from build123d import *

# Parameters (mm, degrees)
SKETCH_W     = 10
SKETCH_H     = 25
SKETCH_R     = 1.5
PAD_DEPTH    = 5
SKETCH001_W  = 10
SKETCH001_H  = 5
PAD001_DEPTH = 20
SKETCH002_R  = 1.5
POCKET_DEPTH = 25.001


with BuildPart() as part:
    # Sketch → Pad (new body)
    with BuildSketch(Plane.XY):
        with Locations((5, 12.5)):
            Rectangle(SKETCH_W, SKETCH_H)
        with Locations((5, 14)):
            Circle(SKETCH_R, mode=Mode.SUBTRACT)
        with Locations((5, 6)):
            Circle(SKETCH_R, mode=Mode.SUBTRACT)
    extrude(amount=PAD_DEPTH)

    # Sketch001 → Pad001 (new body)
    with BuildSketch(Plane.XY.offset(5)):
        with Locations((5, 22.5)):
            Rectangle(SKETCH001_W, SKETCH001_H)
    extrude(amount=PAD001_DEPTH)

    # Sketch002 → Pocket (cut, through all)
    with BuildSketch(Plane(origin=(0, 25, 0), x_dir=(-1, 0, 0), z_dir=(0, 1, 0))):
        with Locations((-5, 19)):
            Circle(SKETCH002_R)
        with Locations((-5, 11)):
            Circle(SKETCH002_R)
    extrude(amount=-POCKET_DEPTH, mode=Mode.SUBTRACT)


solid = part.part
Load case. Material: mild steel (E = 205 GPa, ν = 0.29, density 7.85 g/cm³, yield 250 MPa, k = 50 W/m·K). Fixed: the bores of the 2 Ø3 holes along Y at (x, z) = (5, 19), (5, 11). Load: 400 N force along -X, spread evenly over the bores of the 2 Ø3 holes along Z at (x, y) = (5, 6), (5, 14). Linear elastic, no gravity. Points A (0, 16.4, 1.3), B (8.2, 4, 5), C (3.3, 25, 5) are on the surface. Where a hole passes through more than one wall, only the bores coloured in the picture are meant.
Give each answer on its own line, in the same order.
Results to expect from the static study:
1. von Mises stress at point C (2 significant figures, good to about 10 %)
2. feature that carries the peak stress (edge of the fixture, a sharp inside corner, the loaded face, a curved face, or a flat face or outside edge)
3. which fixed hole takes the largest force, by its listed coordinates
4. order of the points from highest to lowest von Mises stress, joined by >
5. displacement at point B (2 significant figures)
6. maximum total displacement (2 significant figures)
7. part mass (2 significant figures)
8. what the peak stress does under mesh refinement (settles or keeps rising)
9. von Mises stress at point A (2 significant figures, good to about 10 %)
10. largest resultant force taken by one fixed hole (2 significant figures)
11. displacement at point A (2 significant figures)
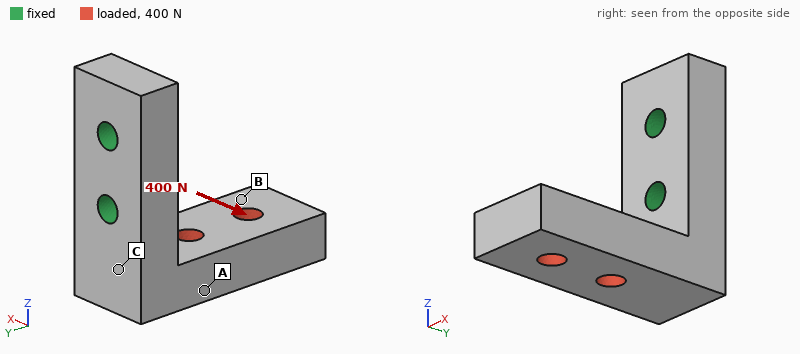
65 MPa
edge of the fixture
(5, 11)
C > A > B
34 µm
41 µm
17 g
keeps rising
33 MPa
590 N
14 µm
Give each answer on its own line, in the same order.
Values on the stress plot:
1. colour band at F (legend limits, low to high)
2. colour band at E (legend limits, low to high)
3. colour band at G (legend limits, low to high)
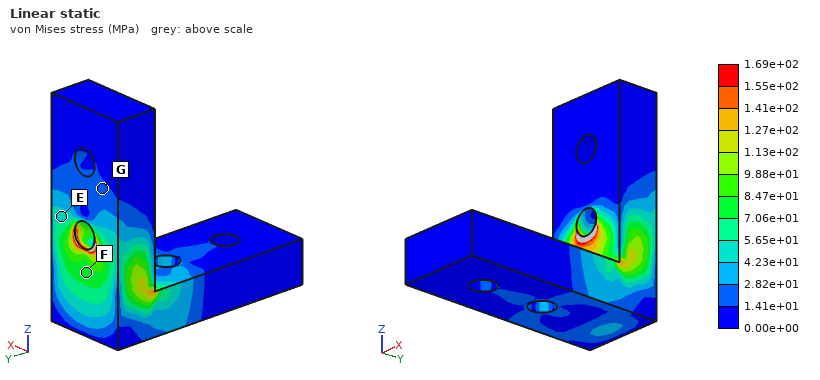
7.06e+01 to 8.47e+01 MPa
4.23e+01 to 5.65e+01 MPa
1.41e+01 to 2.82e+01 MPa
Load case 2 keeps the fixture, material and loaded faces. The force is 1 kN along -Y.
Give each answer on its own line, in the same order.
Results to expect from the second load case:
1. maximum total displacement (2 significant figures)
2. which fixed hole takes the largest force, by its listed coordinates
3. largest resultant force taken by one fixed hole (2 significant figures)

42 µm
(5, 11)
1.2 kN
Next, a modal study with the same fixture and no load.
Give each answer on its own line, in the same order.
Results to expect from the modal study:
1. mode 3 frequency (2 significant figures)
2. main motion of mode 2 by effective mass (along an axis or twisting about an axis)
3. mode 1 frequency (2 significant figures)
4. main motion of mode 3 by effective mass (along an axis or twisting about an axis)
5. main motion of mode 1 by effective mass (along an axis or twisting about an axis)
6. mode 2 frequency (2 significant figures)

19 kHz
along X
5300 Hz
along Y
along Z
6900 Hz
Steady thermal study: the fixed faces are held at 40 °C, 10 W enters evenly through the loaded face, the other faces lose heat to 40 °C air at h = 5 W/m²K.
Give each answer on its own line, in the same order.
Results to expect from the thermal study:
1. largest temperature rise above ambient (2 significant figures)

81 K
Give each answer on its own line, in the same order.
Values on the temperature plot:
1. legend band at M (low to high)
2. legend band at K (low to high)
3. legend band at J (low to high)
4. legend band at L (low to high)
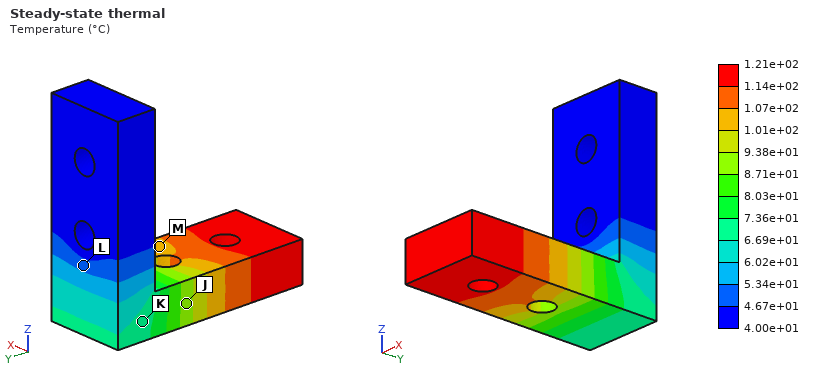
1.01e+02 to 1.07e+02 °C
6.69e+01 to 7.36e+01 °C
8.71e+01 to 9.38e+01 °C
4.67e+01 to 5.34e+01 °C
